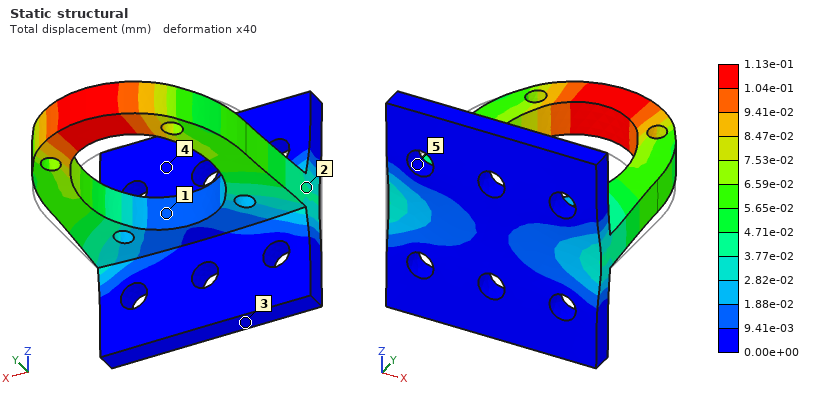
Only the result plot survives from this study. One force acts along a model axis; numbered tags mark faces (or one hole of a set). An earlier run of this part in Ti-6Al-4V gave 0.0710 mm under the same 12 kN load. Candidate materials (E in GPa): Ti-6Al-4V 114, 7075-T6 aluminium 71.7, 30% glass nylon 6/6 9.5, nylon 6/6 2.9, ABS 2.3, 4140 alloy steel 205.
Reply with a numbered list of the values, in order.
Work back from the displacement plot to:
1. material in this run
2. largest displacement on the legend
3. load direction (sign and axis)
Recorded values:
1. 7075-T6 aluminium
2. 1.13e-01 mm
3. +Y
